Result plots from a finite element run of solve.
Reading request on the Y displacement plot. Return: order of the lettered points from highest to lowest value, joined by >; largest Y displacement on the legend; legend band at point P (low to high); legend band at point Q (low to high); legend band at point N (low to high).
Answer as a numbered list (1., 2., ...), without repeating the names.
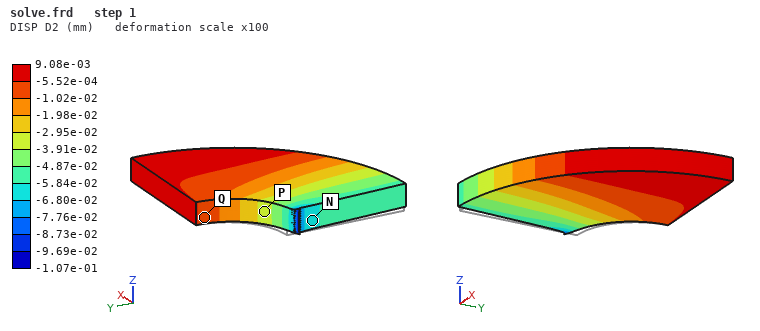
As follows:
1. Q > P > N
2. 9.08e-03 mm
3. -3.91e-02 to -2.95e-02 mm
4. -1.02e-02 to -5.52e-04 mm
5. -6.80e-02 to -5.84e-02 mm
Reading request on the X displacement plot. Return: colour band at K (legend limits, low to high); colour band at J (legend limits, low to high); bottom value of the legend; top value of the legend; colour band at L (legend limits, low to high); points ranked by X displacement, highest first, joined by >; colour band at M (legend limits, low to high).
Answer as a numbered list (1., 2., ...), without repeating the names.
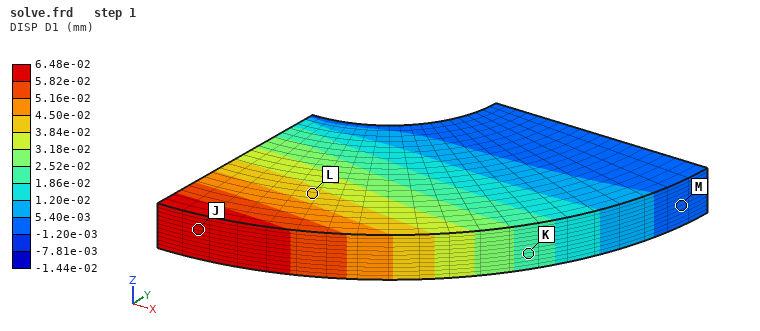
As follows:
1. 1.86e-02 to 2.52e-02 mm
2. 5.82e-02 to 6.48e-02 mm
3. -1.44e-02 mm
4. 6.48e-02 mm
5. 3.84e-02 to 4.50e-02 mm
6. J > L > K > M
7. -1.20e-03 to 5.40e-03 mm
